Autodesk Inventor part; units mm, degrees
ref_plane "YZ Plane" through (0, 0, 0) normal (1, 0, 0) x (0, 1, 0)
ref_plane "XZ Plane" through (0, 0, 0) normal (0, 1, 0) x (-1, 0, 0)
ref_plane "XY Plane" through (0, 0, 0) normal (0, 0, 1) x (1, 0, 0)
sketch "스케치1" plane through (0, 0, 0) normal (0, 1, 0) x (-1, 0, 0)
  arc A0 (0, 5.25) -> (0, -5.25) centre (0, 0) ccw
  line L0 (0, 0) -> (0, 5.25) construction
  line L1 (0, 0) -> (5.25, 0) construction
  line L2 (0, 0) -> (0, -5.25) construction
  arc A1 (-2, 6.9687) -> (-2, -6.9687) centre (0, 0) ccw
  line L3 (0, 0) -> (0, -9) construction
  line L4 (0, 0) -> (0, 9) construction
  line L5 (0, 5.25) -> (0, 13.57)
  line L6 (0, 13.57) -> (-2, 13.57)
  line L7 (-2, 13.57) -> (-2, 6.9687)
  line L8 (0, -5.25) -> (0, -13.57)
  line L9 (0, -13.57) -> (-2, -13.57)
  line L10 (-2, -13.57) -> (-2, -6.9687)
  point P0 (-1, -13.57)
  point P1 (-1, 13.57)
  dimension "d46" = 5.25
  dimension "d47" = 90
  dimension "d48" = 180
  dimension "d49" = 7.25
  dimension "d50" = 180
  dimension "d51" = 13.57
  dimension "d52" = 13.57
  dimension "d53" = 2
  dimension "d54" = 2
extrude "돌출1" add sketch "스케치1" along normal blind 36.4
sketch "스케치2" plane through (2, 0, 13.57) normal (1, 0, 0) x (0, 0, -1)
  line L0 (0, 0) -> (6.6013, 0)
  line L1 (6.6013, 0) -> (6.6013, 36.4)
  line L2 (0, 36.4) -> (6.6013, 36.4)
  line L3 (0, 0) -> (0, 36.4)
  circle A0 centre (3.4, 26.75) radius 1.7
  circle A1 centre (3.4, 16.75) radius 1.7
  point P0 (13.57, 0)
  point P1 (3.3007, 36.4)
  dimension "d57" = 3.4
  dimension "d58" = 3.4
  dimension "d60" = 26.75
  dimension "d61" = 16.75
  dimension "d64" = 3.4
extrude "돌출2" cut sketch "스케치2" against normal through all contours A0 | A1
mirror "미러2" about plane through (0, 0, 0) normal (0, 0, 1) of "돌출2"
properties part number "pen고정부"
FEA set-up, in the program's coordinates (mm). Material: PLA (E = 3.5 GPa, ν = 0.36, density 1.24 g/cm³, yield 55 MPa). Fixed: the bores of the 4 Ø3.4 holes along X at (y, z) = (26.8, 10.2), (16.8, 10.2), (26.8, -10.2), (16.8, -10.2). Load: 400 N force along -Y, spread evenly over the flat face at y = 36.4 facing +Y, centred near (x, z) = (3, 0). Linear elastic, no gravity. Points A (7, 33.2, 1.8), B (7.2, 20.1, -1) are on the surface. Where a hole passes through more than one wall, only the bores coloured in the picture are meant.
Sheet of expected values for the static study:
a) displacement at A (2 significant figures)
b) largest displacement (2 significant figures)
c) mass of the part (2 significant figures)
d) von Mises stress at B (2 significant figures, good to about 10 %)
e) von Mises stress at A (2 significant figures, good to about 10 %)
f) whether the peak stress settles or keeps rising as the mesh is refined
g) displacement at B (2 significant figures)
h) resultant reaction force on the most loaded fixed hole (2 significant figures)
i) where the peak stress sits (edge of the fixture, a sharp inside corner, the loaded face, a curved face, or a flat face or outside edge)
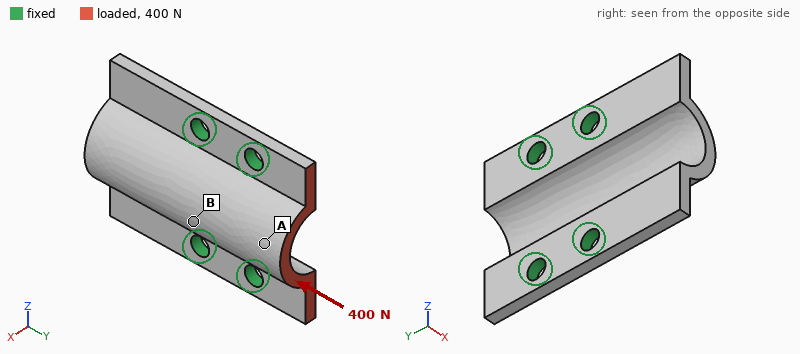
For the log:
71 µm
90 µm
2.8 g
2.6 MPa
7.2 MPa
keeps rising
31 µm
150 N
edge of the fixture
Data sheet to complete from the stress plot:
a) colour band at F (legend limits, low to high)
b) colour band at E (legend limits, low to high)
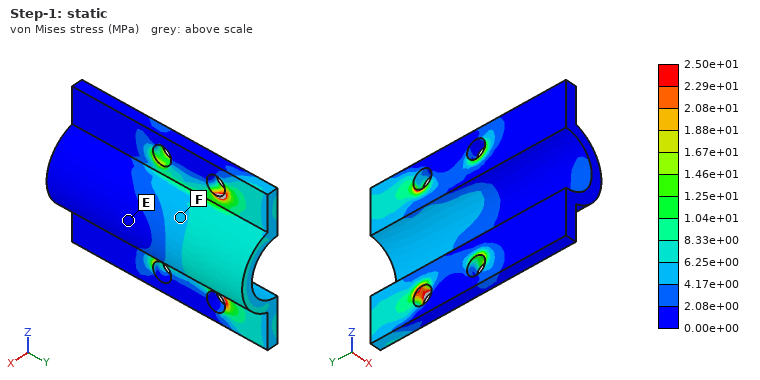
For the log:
4.17e+00 to 6.25e+00 MPa
0.00e+00 to 2.08e+00 MPa
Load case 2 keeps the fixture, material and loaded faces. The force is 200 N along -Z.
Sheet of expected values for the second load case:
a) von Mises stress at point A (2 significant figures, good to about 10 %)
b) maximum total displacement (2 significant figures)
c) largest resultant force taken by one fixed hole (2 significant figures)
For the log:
7.7 MPa
0.14 mm
120 N
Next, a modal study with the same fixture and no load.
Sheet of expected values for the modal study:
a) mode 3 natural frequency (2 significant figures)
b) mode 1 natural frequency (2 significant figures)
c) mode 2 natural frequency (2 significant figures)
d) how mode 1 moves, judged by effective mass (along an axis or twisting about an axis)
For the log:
6600 Hz
3500 Hz
4300 Hz
along X
